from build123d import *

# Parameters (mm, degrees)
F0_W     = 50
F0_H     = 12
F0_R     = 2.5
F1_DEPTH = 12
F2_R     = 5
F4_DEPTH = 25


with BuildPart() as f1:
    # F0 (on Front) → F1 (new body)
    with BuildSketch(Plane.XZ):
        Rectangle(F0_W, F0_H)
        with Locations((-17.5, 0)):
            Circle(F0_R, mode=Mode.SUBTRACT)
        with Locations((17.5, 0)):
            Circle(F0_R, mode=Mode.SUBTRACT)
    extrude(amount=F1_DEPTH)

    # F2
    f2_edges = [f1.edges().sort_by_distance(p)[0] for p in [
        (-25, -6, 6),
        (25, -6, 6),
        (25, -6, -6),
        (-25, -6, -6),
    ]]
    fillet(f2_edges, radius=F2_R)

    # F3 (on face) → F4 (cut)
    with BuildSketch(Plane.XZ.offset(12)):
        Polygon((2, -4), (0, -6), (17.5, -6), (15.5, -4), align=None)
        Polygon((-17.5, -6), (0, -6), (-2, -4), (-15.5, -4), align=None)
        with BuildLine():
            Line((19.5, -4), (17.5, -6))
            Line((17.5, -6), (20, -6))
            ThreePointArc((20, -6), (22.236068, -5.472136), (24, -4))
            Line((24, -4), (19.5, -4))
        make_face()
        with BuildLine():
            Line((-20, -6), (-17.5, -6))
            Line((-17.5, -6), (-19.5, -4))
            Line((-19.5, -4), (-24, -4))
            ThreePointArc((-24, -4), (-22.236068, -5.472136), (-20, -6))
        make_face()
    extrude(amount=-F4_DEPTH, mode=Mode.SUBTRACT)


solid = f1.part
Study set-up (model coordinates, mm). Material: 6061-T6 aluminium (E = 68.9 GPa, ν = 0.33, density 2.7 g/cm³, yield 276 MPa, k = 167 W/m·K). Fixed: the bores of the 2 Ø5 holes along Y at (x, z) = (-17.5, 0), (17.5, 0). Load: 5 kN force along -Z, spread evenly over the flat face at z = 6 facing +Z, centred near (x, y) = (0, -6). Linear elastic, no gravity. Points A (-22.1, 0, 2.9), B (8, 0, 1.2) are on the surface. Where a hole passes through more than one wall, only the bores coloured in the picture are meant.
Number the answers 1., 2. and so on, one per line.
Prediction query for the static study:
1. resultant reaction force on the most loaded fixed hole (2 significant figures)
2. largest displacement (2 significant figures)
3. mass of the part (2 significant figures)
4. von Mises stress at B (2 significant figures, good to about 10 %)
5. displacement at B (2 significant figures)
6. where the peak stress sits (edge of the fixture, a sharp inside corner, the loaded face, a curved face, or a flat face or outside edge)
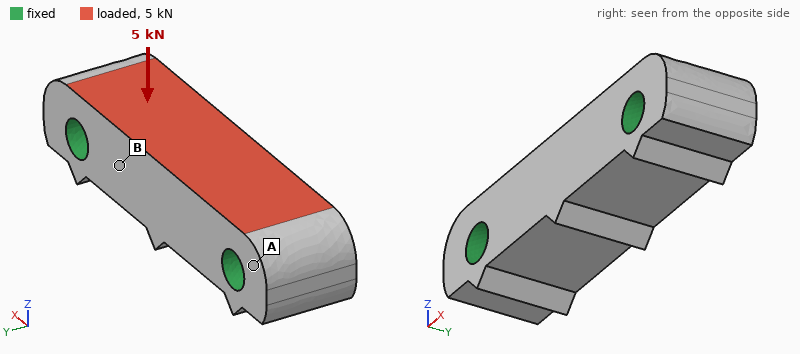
1. 2.5 kN
2. 14 µm
3. 15 g
4. 25 MPa
5. 9.0 µm
6. edge of the fixture
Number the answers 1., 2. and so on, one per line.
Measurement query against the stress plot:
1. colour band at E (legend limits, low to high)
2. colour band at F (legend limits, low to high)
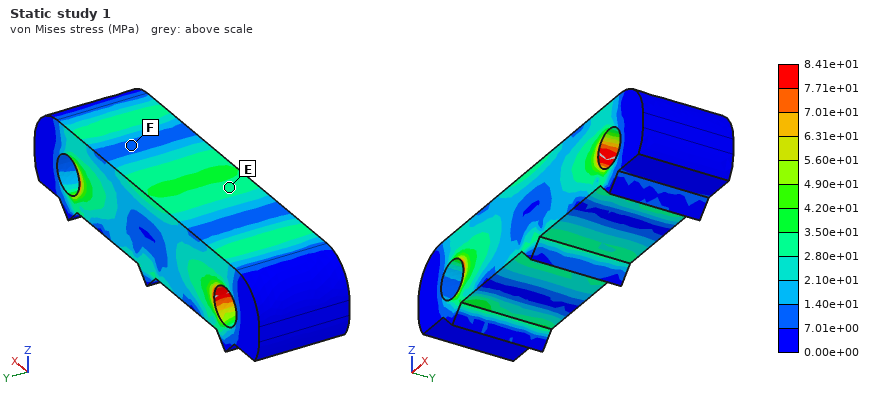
1. 2.80e+01 to 3.50e+01 MPa
2. 7.01e+00 to 1.40e+01 MPa
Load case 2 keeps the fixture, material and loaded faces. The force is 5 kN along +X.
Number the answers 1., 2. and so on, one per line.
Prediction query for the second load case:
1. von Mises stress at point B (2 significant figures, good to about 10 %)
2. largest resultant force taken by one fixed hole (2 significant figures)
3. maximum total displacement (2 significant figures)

1. 13 MPa
2. 2.6 kN
3. 3.6 µm
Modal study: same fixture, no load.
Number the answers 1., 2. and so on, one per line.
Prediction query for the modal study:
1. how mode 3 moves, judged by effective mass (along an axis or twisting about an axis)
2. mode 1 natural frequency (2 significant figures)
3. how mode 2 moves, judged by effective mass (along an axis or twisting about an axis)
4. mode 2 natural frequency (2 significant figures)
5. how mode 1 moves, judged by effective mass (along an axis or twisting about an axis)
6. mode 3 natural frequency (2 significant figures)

1. twisting about X
2. 30 kHz
3. along Y
4. 35 kHz
5. along Z
6. 43 kHz
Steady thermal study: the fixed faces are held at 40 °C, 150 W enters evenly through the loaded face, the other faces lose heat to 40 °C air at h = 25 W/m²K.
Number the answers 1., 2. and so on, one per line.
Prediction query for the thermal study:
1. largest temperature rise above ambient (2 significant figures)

1. 31 K
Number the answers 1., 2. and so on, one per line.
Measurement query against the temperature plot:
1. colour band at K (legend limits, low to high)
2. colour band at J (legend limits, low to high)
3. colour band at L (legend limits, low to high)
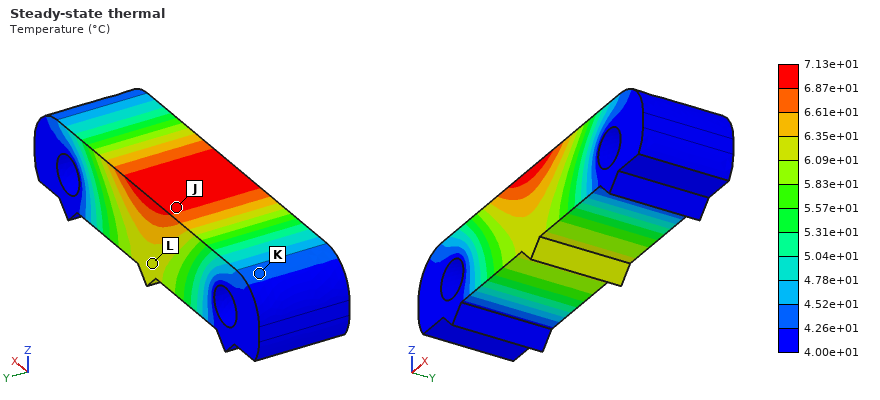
1. 4.26e+01 to 4.52e+01 °C
2. 6.87e+01 to 7.13e+01 °C
3. 6.09e+01 to 6.35e+01 °C
